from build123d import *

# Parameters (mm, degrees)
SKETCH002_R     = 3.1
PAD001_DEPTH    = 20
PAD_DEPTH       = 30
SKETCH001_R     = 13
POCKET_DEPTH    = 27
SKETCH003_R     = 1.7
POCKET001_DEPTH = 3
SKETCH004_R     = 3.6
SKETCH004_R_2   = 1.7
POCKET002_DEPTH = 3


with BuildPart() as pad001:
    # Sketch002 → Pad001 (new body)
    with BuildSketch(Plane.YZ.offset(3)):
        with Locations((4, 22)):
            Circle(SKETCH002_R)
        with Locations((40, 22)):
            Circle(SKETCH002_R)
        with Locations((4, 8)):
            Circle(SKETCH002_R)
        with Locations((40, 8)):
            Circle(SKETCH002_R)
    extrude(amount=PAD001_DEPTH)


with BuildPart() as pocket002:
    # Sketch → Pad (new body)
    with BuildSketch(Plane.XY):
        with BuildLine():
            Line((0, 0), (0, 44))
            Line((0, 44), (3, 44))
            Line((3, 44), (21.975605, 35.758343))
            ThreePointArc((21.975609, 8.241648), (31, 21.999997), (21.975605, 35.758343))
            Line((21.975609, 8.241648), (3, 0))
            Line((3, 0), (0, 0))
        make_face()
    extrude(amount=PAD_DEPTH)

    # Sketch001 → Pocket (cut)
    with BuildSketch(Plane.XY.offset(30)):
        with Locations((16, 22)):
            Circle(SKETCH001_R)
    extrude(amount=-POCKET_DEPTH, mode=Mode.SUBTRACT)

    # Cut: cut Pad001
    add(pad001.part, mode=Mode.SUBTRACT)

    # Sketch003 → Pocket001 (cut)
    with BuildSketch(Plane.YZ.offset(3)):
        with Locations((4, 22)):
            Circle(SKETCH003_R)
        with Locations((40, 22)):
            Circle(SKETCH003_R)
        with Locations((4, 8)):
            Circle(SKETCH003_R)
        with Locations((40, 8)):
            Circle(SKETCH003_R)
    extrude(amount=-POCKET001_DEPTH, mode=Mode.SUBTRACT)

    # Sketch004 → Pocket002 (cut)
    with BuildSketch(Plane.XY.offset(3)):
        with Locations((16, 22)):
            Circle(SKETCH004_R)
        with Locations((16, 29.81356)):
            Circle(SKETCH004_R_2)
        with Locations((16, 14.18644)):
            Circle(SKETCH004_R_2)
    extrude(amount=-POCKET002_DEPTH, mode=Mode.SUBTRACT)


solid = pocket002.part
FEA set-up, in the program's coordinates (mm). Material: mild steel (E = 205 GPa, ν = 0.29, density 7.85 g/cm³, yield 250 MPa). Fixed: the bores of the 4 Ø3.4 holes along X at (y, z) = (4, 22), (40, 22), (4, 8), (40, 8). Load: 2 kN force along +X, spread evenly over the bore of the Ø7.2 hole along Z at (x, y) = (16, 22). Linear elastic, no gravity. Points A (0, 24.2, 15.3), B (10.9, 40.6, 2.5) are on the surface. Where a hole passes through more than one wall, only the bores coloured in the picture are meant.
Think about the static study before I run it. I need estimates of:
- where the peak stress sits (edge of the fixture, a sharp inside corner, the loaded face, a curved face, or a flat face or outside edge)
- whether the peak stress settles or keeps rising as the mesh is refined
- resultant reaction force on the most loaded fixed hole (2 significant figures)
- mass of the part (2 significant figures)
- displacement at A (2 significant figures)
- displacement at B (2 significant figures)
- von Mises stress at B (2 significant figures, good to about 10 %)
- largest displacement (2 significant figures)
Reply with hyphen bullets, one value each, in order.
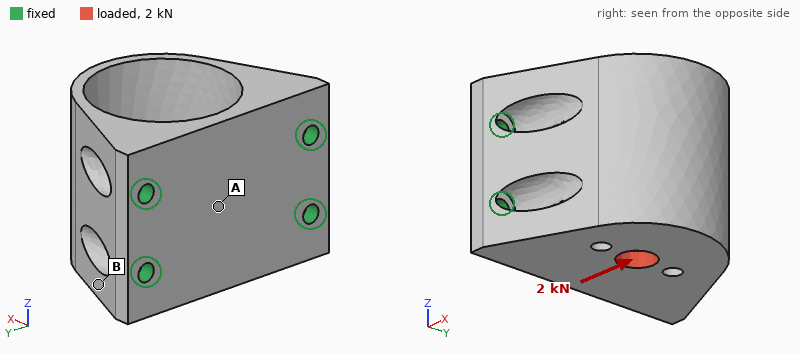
- edge of the fixture
- keeps rising
- 1.4 kN
- 110 g
- 1.5 µm
- 3.6 µm
- 24 MPa
- 9.1 µm
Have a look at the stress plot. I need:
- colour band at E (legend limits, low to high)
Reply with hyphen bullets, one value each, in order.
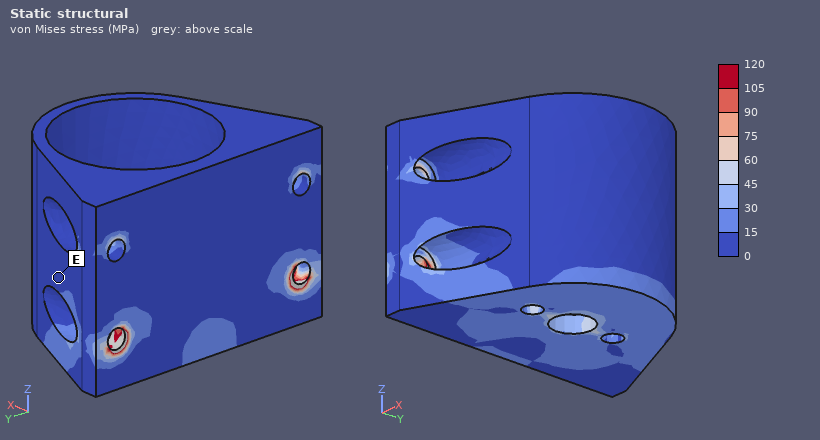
- 0 to 15 MPa
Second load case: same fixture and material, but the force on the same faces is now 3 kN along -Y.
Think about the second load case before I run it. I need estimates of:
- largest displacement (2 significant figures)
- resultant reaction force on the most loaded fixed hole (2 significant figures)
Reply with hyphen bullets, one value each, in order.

- 9.6 µm
- 1.6 kN
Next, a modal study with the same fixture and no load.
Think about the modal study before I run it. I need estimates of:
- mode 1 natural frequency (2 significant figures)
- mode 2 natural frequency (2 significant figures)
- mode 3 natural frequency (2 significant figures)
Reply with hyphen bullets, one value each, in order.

- 10 kHz
- 10 kHz
- 13 kHz
